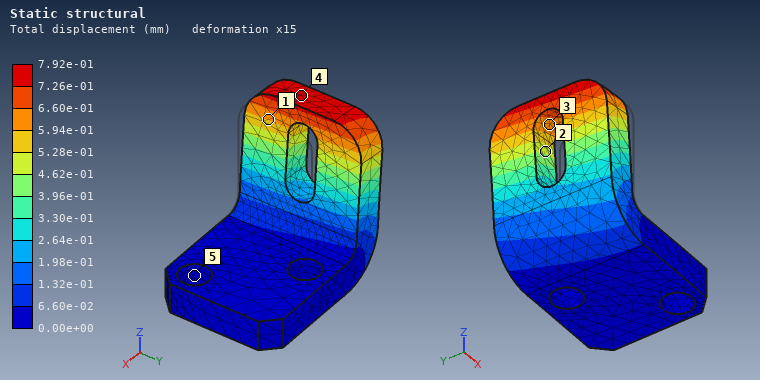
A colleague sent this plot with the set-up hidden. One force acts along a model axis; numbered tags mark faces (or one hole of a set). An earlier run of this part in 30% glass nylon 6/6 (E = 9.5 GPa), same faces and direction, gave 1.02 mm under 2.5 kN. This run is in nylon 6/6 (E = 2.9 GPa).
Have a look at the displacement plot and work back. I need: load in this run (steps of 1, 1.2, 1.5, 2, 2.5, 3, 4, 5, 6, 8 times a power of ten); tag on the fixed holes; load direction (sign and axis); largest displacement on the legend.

600 N
5
-X
7.92e-01 mm
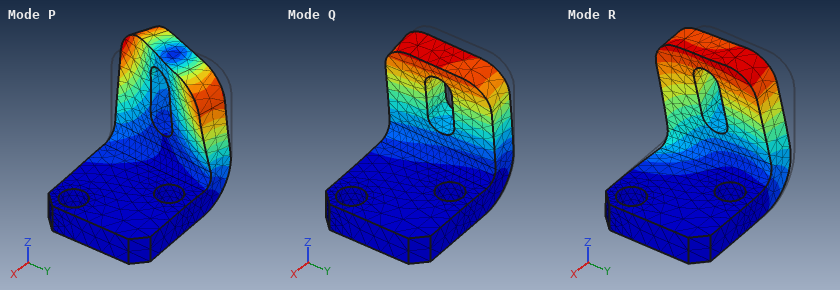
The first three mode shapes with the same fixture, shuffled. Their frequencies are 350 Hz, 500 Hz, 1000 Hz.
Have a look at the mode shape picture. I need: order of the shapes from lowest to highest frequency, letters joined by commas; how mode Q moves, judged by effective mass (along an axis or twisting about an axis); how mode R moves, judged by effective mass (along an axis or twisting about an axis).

Q, R, P
along X
along Y
